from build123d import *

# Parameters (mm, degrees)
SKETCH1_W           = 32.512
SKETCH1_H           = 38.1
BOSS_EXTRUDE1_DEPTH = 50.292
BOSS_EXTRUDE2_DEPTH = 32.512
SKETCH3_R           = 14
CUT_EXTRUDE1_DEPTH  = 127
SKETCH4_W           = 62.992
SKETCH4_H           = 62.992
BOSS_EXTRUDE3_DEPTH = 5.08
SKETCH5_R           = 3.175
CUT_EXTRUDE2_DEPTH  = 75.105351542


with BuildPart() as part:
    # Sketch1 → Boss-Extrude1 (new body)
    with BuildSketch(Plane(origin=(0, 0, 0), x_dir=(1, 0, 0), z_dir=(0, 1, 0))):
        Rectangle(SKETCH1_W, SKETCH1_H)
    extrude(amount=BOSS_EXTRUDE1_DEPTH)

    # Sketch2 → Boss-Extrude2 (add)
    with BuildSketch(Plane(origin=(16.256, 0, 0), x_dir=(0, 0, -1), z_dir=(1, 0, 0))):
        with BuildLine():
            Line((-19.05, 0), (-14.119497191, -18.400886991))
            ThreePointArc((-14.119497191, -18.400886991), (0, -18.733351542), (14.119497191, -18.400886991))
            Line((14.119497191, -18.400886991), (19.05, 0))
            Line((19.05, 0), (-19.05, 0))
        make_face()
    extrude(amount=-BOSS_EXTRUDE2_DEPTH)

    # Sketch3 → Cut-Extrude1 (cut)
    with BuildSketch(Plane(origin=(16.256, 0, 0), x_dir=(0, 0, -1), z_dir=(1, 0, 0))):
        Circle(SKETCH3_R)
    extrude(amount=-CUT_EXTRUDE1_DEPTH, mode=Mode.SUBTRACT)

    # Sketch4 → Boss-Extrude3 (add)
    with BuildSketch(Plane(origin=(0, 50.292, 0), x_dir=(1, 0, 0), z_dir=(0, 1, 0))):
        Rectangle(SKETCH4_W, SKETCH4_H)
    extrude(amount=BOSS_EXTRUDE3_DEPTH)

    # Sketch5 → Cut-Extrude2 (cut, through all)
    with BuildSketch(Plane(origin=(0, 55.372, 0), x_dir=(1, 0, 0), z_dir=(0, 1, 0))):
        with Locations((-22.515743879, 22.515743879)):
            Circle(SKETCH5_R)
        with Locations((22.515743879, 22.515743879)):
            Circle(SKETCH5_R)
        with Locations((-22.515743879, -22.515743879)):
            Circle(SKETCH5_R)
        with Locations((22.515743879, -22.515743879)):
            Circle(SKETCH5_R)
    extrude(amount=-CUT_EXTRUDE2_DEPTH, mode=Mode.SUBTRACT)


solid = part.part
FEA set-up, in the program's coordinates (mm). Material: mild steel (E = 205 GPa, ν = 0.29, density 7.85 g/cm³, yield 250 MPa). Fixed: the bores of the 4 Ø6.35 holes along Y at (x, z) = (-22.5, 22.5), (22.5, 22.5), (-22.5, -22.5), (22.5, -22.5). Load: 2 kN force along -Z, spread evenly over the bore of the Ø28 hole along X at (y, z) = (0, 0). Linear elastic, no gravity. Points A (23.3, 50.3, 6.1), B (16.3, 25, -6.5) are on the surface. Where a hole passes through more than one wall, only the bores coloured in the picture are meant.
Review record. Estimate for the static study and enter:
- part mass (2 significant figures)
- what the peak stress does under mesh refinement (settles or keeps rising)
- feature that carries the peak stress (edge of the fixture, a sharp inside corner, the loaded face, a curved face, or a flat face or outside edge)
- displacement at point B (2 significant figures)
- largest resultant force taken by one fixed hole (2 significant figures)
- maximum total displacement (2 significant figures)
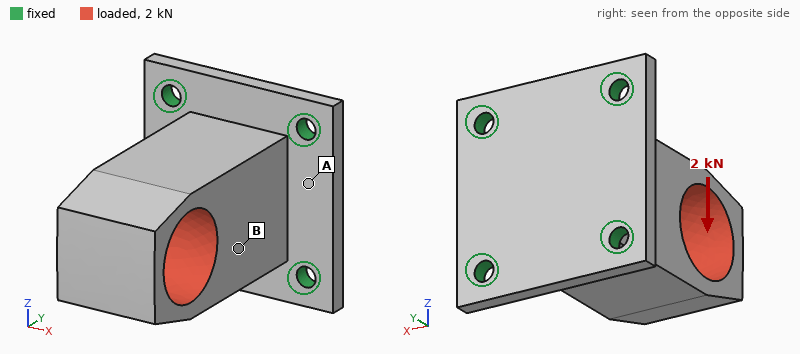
640 g
keeps rising
edge of the fixture
9.4 µm
1.5 kN
32 µm
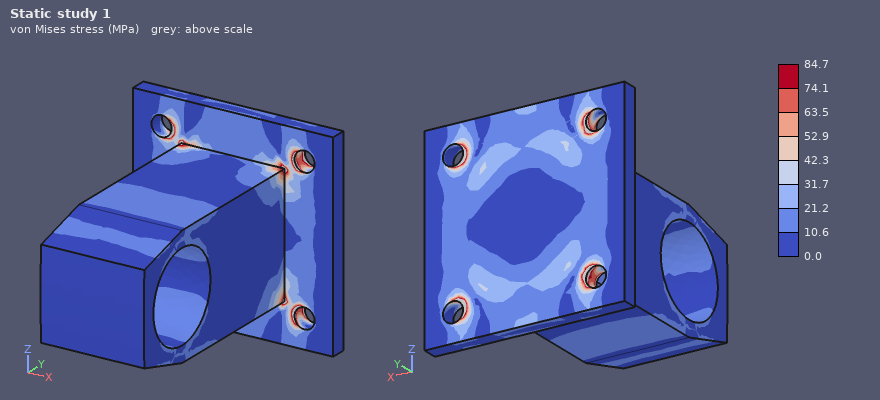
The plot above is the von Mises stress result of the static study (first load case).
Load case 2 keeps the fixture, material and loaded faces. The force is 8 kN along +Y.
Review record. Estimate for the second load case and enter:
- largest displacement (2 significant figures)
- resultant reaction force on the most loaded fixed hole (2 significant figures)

16 µm
2.2 kN
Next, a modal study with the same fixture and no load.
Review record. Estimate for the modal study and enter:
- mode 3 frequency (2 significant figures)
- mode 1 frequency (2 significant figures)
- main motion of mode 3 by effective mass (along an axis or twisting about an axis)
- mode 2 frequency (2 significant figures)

6300 Hz
3100 Hz
along Y
3100 Hz
